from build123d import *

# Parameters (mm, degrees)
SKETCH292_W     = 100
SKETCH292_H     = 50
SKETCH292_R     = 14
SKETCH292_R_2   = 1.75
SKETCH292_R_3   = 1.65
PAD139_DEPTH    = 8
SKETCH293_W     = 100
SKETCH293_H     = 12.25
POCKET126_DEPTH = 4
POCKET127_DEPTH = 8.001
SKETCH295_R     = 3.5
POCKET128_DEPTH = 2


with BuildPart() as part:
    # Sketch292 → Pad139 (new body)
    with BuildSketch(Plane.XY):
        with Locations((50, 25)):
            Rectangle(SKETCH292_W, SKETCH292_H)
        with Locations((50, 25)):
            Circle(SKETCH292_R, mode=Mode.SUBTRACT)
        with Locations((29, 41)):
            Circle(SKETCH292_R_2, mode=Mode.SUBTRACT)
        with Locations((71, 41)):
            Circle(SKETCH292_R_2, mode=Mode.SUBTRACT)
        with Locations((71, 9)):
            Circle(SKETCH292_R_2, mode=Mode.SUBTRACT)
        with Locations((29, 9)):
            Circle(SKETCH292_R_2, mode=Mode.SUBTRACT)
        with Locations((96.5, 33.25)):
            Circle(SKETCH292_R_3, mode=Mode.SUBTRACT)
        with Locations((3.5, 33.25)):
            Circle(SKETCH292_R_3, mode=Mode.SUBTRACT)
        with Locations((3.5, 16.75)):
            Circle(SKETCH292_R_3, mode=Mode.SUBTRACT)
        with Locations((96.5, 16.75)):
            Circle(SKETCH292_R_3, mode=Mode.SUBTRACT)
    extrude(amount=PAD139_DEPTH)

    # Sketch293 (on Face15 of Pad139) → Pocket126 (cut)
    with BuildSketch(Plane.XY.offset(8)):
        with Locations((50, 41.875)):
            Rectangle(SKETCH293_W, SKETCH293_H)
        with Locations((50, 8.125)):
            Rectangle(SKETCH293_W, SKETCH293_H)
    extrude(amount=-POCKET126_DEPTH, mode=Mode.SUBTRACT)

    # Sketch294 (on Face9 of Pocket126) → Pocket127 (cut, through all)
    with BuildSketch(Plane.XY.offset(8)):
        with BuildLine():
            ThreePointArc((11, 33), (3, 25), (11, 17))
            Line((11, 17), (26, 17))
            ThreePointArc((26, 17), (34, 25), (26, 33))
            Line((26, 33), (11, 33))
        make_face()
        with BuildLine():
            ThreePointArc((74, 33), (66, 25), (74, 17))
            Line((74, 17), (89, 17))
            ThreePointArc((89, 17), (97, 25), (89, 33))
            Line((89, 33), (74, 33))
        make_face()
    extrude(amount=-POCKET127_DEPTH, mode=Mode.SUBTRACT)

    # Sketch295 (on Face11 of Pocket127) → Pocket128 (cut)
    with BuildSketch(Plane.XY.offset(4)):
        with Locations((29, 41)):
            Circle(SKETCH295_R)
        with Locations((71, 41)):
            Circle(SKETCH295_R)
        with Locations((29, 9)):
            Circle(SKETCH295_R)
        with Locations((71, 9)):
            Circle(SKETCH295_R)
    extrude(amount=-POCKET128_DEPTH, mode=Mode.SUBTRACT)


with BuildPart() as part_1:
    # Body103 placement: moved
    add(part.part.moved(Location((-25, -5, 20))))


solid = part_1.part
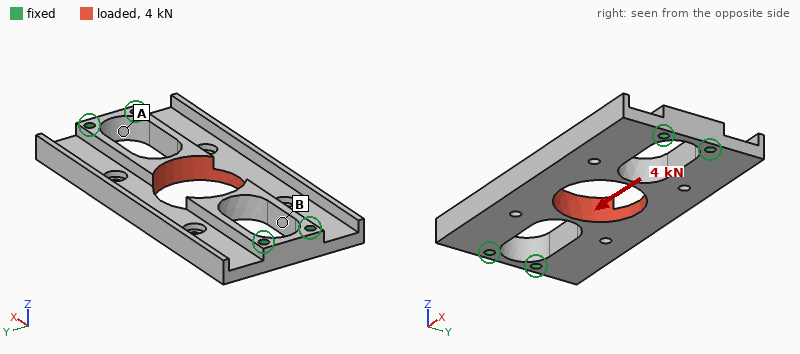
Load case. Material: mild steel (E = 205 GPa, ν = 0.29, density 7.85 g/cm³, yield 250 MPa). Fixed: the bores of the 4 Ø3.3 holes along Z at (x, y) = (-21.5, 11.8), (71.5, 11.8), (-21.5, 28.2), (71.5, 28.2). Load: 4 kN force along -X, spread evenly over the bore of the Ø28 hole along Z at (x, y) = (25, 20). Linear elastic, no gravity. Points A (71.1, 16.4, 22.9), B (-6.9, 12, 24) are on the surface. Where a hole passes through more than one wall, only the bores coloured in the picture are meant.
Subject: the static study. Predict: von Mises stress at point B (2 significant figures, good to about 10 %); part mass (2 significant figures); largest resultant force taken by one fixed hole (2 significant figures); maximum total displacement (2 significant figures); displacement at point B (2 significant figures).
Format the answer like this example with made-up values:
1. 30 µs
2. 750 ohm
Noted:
1. 31 MPa
2. 140 g
3. 1.0 kN
4. 7.3 µm
5. 2.6 µm
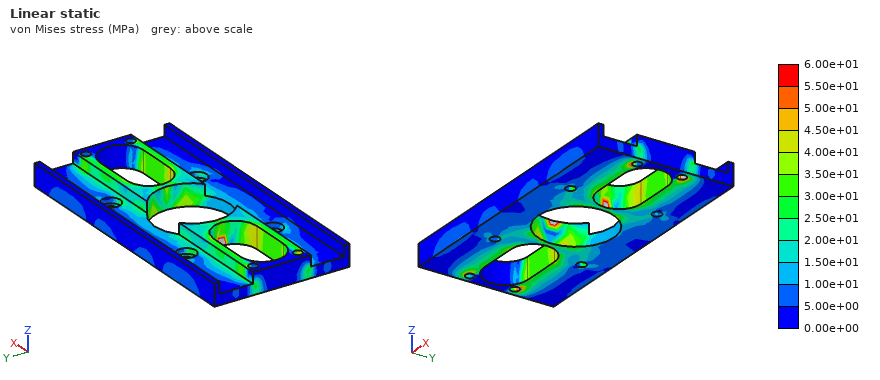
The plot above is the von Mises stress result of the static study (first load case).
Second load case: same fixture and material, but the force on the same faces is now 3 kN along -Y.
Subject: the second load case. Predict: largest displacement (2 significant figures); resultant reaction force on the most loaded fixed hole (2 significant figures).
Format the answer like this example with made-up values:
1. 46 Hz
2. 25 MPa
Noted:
1. 29 µm
2. 1.3 kN
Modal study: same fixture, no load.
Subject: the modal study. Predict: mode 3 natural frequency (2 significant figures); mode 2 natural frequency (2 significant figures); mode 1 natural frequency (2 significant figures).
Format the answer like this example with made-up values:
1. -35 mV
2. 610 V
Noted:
1. 7200 Hz
2. 3200 Hz
3. 3200 Hz
